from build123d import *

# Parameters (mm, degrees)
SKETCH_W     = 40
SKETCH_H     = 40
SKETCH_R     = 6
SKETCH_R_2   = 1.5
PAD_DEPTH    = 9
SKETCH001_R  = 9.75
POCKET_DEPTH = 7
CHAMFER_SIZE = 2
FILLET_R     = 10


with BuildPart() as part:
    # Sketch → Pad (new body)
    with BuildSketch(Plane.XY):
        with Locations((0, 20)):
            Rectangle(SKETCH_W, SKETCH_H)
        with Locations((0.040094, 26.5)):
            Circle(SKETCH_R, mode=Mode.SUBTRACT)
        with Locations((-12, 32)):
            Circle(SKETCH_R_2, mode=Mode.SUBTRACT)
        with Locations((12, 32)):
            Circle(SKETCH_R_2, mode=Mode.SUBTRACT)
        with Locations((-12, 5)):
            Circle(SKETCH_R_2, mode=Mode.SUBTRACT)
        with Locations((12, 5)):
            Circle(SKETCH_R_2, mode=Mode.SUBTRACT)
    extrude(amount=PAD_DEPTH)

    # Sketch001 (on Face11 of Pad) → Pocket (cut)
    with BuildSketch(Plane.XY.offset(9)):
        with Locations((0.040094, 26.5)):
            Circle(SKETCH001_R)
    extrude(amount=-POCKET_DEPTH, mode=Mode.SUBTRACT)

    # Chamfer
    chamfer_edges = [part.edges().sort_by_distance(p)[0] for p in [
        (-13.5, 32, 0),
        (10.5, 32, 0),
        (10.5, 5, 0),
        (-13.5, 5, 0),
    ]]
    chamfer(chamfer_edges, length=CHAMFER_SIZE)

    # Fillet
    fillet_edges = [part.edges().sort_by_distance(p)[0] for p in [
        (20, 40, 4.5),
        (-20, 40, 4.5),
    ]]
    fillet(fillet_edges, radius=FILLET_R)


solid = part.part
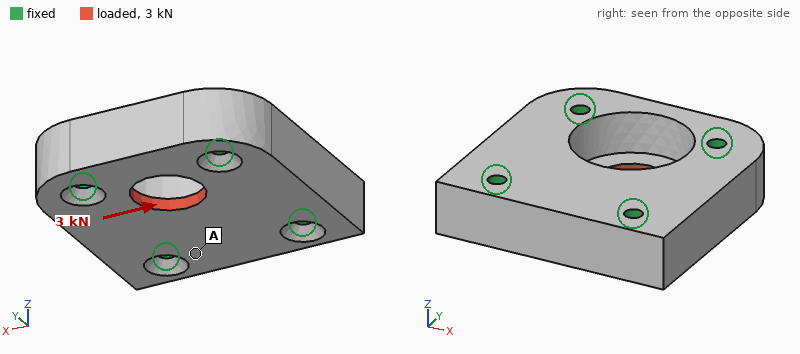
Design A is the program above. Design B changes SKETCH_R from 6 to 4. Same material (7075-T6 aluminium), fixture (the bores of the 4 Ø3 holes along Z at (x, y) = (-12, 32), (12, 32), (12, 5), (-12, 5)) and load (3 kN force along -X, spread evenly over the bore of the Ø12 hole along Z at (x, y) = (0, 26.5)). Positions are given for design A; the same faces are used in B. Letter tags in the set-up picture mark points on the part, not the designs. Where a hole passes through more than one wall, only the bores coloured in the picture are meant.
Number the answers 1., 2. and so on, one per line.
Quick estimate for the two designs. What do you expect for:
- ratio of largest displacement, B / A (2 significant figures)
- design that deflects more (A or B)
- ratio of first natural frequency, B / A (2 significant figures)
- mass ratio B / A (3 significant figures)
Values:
1. 1.1
2. B
3. 0.99
4. 1.01
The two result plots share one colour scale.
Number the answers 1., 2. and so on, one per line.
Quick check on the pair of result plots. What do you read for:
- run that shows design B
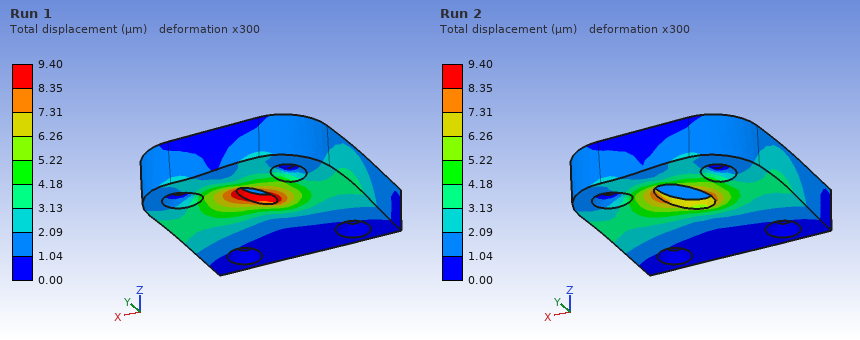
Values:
1. Run 1
